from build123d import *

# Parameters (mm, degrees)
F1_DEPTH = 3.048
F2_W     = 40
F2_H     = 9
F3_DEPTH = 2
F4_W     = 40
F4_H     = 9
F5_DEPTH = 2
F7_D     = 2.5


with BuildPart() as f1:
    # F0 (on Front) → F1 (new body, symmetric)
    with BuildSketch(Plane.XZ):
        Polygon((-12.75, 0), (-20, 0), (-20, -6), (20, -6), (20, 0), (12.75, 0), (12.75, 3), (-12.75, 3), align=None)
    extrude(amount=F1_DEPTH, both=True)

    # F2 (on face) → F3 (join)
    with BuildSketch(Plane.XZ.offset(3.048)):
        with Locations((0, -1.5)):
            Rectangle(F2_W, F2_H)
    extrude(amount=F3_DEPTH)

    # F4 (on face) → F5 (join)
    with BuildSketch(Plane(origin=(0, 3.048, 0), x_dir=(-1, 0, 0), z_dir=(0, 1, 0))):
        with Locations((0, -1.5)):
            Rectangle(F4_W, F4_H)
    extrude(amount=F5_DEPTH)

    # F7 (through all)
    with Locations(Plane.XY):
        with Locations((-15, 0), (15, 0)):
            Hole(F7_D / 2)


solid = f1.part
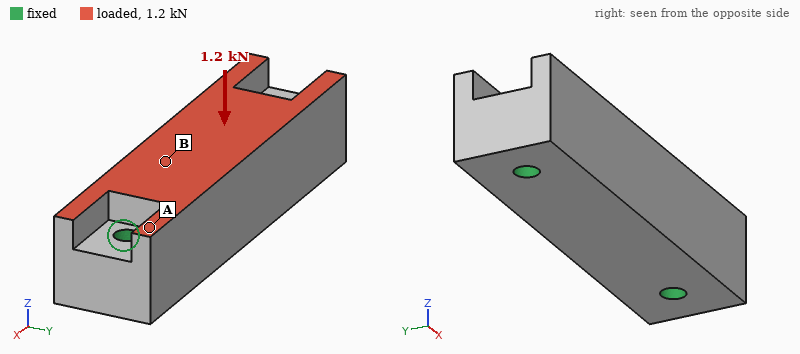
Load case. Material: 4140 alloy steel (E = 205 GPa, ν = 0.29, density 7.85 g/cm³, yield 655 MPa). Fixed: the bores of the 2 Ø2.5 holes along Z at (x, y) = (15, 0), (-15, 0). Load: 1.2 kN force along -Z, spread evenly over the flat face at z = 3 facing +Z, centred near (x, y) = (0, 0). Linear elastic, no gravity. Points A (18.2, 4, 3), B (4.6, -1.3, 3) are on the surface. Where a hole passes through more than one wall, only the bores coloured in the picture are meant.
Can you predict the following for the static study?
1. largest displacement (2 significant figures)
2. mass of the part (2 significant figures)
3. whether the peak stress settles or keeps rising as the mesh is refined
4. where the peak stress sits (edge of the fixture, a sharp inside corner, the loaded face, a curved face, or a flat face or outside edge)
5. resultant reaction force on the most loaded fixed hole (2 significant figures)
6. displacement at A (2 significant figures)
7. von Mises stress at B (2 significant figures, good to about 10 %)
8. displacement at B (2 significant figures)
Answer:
2.0 µm
26 g
keeps rising
edge of the fixture
630 N
0.49 µm
14 MPa
1.8 µm
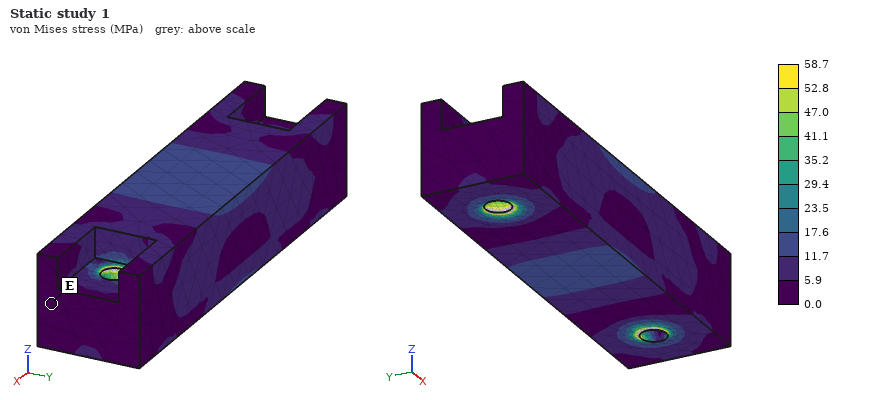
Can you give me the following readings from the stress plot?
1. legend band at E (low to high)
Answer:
0.0 to 5.9 MPa
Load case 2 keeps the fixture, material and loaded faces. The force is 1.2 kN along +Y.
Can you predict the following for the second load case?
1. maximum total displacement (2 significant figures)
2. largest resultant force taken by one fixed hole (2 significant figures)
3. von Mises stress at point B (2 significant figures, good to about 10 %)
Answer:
5.3 µm
600 N
15 MPa
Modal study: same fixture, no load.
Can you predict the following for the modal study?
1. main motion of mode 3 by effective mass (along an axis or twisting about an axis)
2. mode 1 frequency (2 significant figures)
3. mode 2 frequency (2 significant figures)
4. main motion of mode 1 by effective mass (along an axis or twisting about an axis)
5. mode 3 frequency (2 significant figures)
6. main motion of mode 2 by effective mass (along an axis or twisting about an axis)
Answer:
twisting about X
26 kHz
29 kHz
along Y
37 kHz
along Z
